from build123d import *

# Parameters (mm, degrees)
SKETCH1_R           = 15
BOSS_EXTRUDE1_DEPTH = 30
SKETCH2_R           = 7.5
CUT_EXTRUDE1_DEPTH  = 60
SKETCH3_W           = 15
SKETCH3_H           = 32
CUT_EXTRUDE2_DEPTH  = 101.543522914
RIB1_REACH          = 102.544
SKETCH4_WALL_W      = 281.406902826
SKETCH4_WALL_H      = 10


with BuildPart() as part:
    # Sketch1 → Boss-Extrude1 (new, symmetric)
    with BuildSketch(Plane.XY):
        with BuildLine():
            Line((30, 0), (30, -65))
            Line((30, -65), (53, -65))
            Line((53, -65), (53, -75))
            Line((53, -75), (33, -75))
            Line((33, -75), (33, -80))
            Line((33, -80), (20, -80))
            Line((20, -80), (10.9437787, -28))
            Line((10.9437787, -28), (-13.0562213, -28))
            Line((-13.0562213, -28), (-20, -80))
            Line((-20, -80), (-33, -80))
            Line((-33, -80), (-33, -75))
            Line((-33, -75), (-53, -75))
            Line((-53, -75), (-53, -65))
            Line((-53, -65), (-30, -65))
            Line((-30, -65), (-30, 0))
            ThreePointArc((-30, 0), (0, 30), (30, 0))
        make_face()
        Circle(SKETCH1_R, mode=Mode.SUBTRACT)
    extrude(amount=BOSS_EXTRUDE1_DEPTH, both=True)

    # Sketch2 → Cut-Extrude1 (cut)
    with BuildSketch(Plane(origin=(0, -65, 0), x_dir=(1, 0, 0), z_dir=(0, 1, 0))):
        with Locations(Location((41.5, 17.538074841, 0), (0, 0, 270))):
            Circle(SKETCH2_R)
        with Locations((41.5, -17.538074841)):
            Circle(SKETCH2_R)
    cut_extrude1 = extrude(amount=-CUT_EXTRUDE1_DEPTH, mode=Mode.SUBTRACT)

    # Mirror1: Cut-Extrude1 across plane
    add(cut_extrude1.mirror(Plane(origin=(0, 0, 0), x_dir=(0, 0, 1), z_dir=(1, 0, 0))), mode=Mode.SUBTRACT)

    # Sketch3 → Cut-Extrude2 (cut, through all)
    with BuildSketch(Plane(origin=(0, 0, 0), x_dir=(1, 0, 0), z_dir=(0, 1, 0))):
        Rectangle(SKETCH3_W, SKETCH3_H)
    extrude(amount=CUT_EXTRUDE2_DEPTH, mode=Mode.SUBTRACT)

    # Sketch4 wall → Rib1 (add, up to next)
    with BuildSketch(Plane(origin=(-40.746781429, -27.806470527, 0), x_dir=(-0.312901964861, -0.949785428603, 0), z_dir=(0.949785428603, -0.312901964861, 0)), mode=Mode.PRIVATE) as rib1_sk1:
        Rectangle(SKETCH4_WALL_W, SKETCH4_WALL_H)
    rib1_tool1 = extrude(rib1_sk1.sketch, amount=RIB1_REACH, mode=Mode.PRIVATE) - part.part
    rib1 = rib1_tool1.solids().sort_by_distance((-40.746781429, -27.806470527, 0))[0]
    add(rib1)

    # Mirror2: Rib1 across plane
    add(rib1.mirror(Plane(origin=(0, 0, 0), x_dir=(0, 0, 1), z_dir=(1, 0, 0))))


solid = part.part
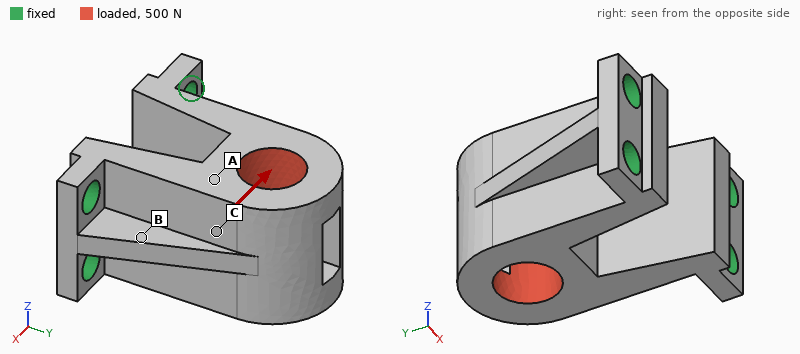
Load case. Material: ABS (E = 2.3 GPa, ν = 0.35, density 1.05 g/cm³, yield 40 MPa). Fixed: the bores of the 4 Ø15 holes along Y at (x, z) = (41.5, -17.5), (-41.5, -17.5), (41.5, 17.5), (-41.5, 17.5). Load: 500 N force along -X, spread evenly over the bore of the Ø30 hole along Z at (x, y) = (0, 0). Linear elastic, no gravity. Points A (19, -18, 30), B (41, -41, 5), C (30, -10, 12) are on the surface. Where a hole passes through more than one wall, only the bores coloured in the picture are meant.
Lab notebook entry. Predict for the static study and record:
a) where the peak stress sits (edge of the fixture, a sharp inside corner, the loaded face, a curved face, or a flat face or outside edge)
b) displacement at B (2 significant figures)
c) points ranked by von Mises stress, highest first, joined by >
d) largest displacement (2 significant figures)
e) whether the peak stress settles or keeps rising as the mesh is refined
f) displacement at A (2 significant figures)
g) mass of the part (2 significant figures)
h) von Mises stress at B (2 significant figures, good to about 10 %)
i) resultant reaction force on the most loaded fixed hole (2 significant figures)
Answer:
edge of the fixture
38 µm
B > A > C
94 µm
keeps rising
60 µm
270 g
0.81 MPa
250 N
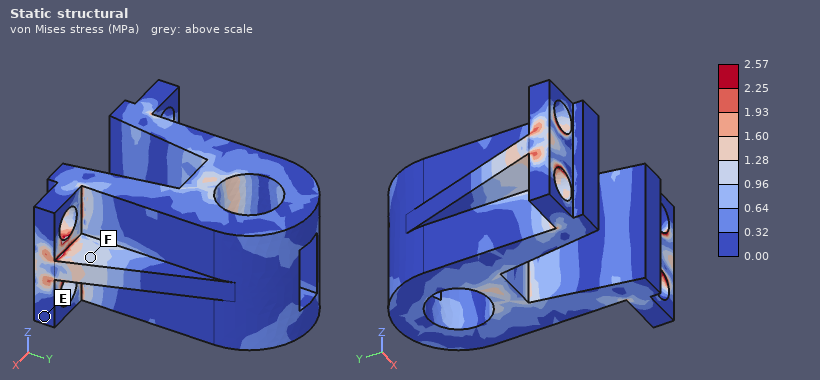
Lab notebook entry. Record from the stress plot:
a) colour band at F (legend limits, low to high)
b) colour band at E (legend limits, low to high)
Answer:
0.96 to 1.28 MPa
0.00 to 0.32 MPa
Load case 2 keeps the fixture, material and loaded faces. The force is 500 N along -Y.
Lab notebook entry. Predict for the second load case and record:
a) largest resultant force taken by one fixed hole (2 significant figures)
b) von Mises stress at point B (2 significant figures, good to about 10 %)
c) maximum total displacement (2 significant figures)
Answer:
130 N
0.38 MPa
15 µm
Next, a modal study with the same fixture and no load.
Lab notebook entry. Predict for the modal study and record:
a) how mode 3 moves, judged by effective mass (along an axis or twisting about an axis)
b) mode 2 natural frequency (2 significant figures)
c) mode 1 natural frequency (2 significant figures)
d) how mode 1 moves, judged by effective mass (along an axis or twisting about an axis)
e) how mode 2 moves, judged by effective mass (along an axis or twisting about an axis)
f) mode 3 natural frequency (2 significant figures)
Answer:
twisting about Y
1000 Hz
670 Hz
along Z
along X
1300 Hz
